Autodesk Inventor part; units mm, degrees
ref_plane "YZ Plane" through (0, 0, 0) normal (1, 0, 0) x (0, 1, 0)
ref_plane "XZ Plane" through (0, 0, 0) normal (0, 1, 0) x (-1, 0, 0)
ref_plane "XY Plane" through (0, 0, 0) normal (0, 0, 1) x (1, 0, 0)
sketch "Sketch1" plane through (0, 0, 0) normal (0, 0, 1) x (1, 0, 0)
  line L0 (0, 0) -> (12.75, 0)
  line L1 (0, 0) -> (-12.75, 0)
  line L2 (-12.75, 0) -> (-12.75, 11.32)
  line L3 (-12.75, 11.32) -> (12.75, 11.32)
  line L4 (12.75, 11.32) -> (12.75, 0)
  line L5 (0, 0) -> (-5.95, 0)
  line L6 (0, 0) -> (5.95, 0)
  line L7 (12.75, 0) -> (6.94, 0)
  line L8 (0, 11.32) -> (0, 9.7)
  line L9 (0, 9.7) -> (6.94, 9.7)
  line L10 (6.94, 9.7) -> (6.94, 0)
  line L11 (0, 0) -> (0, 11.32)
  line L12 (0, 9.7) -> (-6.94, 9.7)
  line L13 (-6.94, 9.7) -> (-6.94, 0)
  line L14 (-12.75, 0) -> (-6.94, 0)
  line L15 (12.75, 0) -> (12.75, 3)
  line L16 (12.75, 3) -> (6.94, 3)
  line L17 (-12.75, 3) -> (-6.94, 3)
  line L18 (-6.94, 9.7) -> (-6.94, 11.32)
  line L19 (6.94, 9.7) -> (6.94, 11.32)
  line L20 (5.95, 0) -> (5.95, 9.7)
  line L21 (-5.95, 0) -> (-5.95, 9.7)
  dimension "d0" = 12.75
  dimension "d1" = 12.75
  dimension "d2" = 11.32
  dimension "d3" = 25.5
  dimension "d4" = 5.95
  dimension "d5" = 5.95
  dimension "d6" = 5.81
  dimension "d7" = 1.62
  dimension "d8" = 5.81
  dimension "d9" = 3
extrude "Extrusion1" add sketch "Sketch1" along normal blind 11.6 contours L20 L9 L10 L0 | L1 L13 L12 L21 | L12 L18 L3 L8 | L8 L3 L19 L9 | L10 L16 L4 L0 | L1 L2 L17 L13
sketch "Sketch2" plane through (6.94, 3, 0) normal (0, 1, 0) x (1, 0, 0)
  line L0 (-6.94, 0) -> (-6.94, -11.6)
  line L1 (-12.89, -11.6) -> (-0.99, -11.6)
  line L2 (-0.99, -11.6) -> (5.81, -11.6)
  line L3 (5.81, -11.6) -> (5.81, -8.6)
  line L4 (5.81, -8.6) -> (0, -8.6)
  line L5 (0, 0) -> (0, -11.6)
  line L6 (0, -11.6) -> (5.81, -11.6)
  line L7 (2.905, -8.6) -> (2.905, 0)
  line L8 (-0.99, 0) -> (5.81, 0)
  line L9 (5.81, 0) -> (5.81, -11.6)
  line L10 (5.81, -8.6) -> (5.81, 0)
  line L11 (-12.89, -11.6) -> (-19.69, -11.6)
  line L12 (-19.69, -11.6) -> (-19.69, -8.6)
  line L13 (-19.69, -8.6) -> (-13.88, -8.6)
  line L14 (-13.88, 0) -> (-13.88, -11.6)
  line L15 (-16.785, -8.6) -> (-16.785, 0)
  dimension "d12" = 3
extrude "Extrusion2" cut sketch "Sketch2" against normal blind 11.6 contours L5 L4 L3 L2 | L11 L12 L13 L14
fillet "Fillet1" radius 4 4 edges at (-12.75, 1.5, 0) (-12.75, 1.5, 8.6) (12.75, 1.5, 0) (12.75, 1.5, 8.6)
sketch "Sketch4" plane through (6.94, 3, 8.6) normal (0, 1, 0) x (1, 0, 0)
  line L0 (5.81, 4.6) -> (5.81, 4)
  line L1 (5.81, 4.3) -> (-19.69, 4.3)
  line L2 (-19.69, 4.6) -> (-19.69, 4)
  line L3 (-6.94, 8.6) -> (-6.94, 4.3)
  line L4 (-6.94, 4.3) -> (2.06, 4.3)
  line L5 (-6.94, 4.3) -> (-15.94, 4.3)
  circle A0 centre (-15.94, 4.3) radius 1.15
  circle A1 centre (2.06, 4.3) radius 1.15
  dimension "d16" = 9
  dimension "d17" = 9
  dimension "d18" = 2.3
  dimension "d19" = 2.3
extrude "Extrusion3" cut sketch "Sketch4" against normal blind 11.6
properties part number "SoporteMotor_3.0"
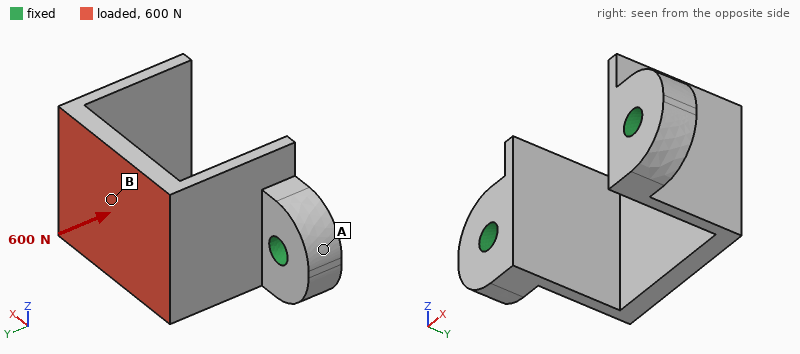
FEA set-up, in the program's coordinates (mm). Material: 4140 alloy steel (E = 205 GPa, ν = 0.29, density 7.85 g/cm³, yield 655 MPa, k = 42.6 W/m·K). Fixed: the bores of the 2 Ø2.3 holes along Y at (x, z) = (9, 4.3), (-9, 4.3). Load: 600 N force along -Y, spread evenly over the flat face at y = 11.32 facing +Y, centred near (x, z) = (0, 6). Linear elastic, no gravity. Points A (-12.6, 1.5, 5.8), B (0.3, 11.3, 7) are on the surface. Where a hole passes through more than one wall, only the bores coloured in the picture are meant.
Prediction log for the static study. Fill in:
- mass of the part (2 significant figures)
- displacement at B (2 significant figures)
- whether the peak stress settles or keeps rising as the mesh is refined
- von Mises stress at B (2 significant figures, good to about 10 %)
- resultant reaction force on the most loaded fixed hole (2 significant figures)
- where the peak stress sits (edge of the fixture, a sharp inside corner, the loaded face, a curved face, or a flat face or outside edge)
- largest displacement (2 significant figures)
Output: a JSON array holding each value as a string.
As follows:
["5.6 g", "13 µm", "keeps rising", "110 MPa", "310 N", "edge of the fixture", "16 µm"]
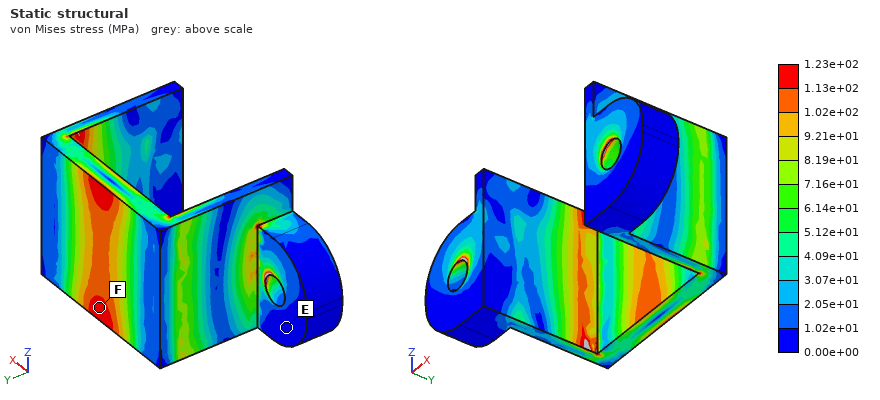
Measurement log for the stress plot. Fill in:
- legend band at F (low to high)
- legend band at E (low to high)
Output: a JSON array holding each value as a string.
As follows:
["1.13e+02 to 1.23e+02 MPa", "0.00e+00 to 1.02e+01 MPa"]
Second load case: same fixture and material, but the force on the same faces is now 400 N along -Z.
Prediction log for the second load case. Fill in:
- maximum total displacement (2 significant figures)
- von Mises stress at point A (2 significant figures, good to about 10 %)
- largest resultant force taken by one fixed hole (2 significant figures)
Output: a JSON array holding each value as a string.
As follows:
["19 µm", "23 MPa", "200 N"]
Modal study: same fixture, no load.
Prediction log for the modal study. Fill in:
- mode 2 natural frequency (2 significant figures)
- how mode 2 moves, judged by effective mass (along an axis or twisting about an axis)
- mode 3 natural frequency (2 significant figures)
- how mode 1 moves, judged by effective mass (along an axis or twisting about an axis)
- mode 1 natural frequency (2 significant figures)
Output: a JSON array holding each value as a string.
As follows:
["16 kHz", "along Z", "21 kHz", "along X", "9100 Hz"]
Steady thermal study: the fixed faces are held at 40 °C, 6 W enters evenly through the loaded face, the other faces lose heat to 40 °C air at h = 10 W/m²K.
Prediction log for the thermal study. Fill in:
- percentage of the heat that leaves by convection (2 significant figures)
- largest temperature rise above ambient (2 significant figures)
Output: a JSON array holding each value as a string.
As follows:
["4.4 %", "66 K"]
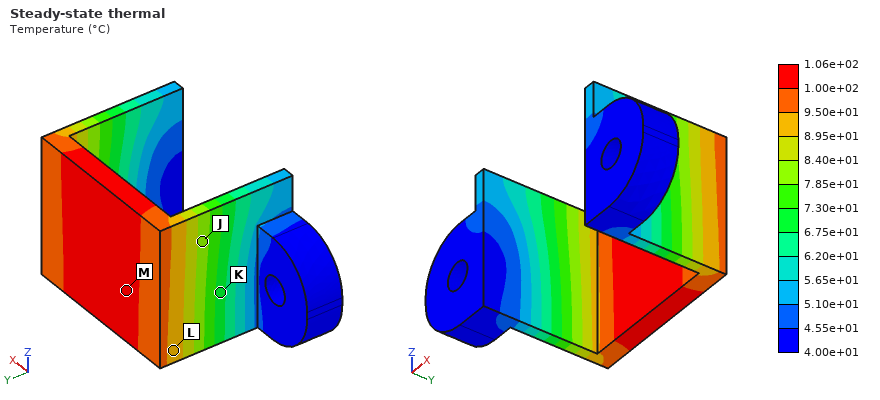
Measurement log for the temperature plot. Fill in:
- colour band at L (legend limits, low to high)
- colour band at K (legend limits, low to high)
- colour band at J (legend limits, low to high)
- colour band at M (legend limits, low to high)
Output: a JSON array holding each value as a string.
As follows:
["8.95e+01 to 9.50e+01 °C", "6.75e+01 to 7.30e+01 °C", "7.85e+01 to 8.40e+01 °C", "1.00e+02 to 1.06e+02 °C"]
